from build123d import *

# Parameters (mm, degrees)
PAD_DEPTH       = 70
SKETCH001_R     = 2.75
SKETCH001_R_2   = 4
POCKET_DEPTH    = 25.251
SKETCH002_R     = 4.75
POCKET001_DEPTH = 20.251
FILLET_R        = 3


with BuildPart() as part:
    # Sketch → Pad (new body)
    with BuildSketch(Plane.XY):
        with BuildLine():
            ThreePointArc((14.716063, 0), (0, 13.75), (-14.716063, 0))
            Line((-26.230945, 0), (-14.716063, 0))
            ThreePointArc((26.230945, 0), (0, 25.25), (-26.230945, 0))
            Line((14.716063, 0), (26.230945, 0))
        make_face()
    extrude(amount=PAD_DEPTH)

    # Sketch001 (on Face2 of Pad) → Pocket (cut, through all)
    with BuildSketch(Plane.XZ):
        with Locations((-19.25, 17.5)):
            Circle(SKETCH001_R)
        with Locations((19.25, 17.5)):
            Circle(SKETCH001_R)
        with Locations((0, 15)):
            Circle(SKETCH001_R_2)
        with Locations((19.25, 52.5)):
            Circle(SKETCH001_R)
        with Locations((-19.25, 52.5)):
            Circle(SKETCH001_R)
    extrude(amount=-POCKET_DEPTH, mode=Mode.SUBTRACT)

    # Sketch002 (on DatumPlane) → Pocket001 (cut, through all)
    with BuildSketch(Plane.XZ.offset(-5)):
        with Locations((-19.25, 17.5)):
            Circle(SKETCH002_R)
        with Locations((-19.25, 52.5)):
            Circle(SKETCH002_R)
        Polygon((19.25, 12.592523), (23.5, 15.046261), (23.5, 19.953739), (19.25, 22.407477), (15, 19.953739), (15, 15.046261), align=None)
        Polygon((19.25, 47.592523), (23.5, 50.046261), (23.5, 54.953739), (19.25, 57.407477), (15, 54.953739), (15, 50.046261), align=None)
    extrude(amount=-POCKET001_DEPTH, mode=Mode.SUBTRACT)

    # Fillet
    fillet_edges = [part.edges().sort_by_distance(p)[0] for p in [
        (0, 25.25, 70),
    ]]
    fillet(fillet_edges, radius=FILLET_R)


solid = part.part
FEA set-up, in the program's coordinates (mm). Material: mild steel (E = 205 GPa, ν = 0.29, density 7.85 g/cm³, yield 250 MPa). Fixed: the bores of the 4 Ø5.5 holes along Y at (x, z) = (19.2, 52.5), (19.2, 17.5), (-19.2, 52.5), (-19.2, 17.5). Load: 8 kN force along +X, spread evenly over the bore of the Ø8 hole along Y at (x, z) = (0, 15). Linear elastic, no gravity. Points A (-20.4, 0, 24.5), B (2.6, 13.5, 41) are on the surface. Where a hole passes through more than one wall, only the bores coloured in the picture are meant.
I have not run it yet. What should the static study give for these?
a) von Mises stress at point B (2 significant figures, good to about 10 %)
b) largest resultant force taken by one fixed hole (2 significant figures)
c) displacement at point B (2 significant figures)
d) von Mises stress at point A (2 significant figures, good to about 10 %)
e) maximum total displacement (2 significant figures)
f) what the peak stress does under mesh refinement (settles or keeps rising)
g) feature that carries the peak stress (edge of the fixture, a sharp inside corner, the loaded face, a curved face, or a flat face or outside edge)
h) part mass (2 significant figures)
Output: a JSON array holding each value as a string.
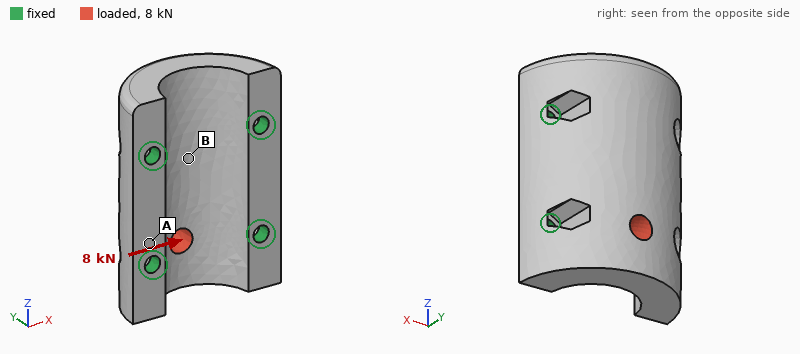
["9.7 MPa", "3.6 kN", "3.1 µm", "23 MPa", "8.7 µm", "keeps rising", "edge of the fixture", "360 g"]
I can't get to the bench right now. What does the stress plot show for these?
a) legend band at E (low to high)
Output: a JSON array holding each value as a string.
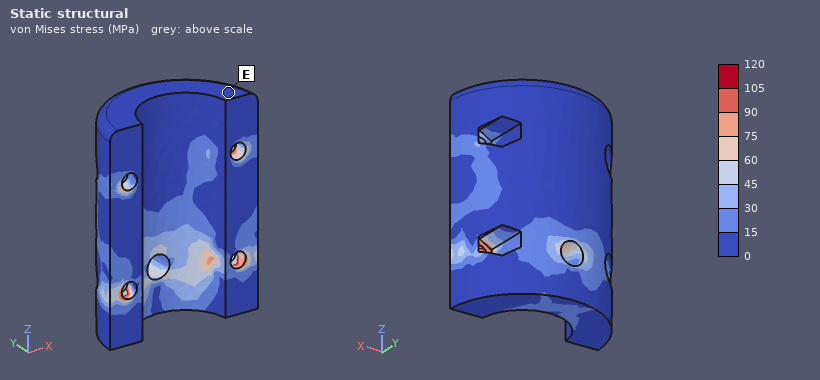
["0 to 15 MPa"]
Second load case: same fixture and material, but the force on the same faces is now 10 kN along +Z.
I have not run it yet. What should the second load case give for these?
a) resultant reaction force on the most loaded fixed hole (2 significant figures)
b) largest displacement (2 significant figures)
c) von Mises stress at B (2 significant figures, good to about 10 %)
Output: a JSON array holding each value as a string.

["3.6 kN", "13 µm", "14 MPa"]
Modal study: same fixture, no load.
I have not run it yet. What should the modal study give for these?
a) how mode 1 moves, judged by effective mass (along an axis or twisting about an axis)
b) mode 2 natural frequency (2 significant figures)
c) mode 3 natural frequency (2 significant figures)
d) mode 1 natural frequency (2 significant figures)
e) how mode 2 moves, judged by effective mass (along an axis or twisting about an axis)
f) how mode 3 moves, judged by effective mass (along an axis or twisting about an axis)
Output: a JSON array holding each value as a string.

["along Z", "13 kHz", "16 kHz", "12 kHz", "along X", "twisting about Y"]
